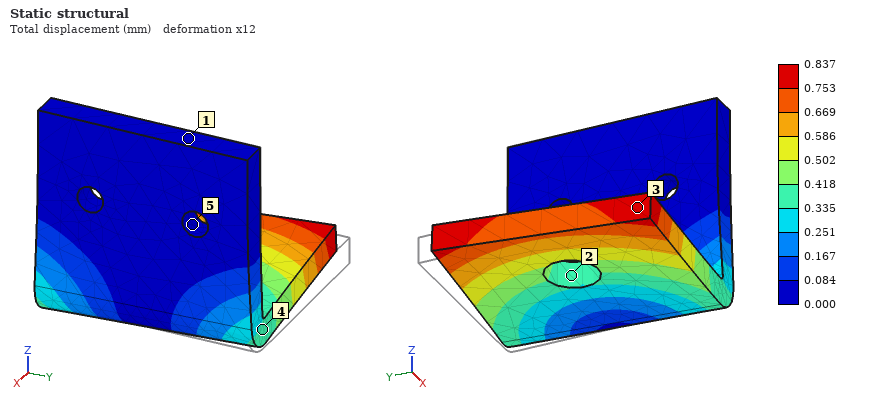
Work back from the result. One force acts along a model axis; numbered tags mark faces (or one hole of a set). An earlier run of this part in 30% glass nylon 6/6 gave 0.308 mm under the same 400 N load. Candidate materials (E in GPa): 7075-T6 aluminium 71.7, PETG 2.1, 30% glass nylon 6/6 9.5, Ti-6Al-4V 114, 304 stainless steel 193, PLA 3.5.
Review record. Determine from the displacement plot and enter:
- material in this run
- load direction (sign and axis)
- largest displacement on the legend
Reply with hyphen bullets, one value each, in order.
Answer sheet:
- PLA
- -Y
- 0.837 mm
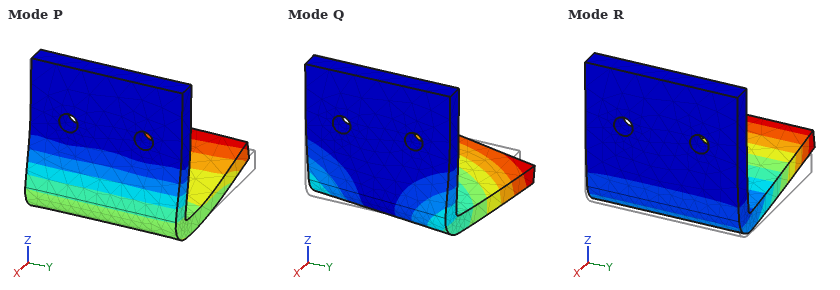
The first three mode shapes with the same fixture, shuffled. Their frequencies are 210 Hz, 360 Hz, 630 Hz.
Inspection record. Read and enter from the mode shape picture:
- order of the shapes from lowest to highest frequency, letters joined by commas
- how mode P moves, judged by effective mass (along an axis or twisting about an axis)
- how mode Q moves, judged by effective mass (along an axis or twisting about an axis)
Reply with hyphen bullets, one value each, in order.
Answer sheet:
- R, Q, P
- along X
- along Y
